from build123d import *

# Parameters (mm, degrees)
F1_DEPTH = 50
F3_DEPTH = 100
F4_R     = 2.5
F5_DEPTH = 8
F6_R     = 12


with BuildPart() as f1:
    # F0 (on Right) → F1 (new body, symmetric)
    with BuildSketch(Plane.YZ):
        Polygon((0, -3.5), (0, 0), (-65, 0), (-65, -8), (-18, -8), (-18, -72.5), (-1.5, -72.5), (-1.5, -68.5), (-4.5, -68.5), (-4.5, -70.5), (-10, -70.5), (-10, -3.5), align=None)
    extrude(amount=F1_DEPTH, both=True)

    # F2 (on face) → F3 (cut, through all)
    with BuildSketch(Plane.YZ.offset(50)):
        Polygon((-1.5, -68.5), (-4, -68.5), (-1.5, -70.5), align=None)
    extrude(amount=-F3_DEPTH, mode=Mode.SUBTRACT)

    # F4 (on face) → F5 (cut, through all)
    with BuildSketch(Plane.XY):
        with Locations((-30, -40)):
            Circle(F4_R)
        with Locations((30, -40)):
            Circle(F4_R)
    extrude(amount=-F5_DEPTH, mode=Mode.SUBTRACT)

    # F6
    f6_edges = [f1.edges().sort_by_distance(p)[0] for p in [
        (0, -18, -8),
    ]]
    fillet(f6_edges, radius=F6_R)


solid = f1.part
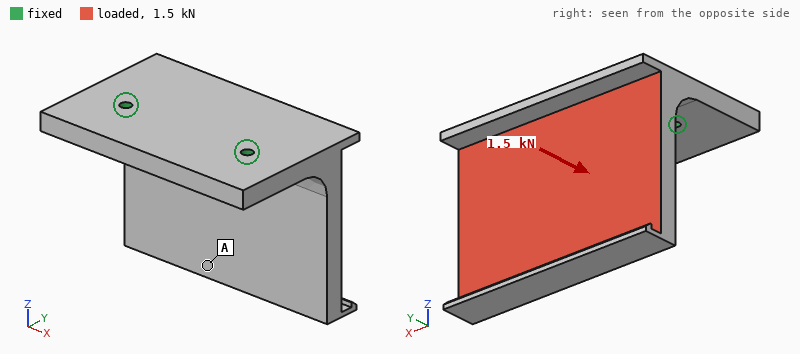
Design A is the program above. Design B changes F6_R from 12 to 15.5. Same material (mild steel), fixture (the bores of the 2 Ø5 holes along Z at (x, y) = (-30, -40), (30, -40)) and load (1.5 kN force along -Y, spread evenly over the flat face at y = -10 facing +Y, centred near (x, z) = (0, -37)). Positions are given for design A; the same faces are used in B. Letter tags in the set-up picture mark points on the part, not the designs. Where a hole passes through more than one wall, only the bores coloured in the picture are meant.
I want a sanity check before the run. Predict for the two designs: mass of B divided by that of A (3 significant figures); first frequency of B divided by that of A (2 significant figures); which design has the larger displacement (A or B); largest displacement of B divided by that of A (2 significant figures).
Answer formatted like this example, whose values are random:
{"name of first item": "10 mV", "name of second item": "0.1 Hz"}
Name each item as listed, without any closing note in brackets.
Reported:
{"mass of B divided by that of A": "1.02", "first frequency of B divided by that of A": "1.0", "which design has the larger displacement": "A", "largest displacement of B divided by that of A": "0.89"}
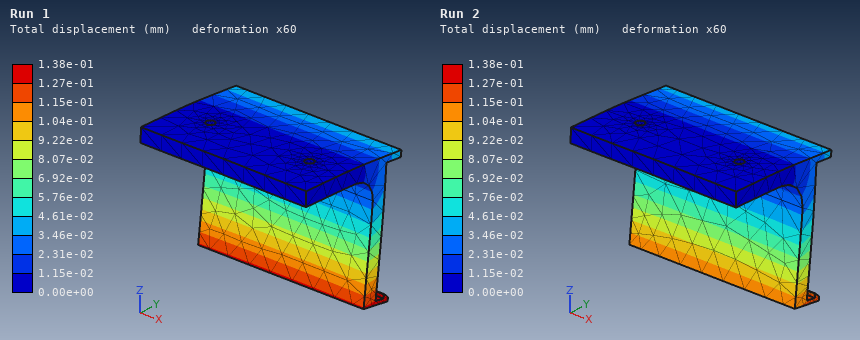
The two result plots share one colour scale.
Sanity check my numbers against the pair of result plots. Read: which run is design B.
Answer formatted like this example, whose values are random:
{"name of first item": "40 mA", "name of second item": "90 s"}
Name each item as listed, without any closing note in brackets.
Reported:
{"which run is design B": "Run 2"}
